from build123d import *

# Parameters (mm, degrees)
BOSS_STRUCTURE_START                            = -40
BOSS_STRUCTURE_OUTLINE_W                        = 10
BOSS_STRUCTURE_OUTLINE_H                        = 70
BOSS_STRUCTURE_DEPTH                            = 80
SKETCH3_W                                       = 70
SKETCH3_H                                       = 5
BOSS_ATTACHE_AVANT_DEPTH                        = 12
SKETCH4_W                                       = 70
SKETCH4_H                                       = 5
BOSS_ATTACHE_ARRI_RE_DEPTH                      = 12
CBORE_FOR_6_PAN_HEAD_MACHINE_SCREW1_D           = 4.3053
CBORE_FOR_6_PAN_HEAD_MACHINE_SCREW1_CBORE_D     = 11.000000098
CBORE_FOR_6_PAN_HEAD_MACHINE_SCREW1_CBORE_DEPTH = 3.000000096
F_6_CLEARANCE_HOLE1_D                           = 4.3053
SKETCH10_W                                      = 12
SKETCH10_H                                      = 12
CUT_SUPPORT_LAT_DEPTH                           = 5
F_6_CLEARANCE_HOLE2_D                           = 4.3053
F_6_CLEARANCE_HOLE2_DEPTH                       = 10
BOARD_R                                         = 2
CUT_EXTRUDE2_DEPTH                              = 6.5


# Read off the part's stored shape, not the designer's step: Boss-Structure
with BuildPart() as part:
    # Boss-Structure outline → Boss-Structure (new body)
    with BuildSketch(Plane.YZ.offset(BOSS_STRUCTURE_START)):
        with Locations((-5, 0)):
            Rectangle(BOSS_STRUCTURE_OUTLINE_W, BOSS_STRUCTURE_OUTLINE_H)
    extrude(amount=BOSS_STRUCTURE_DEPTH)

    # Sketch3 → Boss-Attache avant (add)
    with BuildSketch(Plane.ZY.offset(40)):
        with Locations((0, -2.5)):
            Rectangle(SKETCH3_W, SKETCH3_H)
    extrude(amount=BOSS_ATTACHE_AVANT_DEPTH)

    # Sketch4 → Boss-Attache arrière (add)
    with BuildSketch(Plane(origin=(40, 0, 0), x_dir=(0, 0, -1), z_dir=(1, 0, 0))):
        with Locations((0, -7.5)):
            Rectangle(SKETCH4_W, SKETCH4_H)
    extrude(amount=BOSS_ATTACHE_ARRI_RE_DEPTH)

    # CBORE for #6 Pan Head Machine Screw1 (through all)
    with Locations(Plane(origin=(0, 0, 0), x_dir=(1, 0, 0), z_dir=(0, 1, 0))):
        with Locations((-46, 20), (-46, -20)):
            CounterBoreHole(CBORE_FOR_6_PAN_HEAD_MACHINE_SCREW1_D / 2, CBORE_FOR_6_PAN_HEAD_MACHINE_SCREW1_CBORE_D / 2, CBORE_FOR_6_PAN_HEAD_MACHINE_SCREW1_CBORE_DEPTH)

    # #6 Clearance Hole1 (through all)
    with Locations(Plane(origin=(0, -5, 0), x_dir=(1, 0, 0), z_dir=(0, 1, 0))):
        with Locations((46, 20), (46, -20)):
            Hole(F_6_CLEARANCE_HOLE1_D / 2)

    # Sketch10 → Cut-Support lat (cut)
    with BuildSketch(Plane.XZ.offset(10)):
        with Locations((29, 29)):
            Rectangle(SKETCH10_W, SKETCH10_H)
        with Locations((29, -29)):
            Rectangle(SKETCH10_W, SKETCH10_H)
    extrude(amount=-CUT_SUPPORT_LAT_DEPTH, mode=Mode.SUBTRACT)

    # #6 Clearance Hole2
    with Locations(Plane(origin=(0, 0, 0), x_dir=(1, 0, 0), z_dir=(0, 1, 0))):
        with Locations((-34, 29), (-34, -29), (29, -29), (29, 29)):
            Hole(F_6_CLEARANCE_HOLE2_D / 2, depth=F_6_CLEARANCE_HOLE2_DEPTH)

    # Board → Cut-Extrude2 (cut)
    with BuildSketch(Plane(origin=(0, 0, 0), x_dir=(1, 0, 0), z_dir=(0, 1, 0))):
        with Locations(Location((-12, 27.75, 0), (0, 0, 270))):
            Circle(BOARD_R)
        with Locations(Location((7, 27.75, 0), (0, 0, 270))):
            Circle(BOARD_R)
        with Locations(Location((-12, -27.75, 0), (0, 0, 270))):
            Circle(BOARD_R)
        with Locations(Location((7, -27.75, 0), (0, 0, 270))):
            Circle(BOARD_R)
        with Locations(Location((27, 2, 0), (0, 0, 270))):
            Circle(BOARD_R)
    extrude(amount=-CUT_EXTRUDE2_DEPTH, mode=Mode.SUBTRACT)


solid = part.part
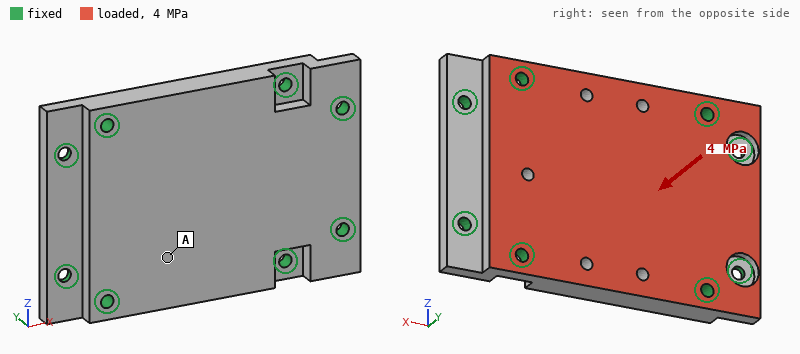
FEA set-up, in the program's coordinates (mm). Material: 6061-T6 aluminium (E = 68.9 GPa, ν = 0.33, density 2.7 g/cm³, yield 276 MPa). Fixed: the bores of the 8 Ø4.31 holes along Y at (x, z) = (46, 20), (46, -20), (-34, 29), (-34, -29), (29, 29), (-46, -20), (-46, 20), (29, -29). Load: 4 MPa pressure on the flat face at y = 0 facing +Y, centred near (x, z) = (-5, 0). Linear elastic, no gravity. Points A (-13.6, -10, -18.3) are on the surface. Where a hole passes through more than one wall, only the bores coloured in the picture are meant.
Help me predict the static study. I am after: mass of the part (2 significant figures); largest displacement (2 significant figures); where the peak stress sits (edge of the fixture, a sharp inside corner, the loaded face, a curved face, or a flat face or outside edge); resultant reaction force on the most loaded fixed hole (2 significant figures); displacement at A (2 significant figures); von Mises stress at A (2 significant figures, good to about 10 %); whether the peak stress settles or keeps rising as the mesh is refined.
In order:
170 g
97 µm
edge of the fixture
5.9 kN
71 µm
40 MPa
keeps rising
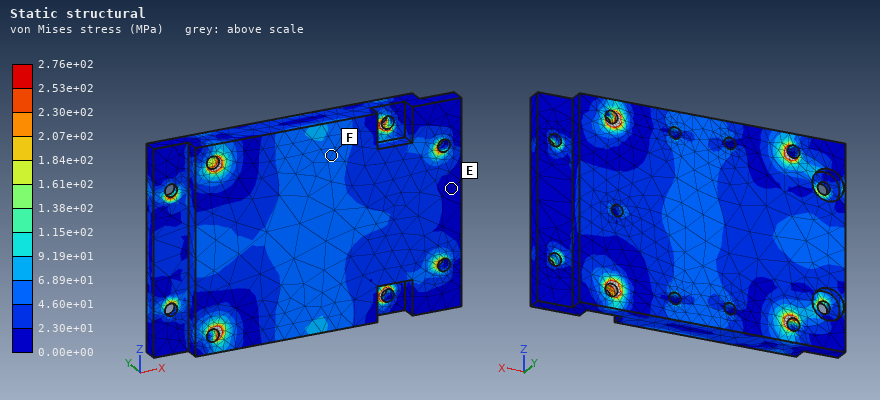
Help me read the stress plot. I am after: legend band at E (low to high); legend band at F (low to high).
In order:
0.00e+00 to 2.30e+01 MPa
4.60e+01 to 6.89e+01 MPa
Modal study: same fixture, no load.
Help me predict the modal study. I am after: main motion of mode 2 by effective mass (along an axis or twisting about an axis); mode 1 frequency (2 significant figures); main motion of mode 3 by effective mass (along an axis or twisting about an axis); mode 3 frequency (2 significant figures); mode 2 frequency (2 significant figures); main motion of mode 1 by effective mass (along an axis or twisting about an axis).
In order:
twisting about X
7300 Hz
twisting about Z
13 kHz
11 kHz
along Y
